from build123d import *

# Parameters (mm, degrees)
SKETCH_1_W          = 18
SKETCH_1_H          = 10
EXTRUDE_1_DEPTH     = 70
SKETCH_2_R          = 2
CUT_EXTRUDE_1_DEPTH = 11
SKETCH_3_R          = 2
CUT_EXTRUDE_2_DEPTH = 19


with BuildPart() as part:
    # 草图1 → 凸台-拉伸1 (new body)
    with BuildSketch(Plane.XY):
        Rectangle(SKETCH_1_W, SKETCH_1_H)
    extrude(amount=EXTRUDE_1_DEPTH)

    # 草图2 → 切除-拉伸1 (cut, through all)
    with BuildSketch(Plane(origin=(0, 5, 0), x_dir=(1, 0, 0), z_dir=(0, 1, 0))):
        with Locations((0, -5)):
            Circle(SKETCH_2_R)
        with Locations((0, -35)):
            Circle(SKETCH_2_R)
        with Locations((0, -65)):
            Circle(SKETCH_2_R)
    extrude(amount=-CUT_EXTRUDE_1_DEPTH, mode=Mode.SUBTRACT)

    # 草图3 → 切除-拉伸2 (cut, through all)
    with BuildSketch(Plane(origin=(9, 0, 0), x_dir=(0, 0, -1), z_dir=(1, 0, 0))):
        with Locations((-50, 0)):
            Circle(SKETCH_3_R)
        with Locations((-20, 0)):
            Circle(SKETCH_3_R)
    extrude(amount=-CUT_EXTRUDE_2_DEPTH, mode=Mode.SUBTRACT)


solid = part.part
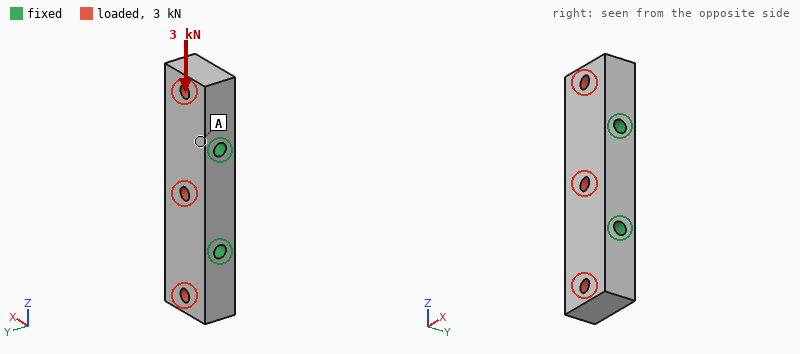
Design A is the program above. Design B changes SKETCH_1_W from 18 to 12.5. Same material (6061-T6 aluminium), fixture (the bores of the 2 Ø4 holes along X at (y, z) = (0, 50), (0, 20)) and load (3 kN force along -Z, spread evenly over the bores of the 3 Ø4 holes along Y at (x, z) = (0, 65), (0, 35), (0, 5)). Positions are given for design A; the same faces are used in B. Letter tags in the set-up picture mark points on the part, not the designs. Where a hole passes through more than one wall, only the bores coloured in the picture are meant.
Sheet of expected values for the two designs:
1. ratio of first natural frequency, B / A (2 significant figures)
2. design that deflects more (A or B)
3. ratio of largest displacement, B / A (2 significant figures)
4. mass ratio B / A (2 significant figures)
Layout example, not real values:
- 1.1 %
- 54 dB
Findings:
- 1.0
- B
- 1.2
- 0.68
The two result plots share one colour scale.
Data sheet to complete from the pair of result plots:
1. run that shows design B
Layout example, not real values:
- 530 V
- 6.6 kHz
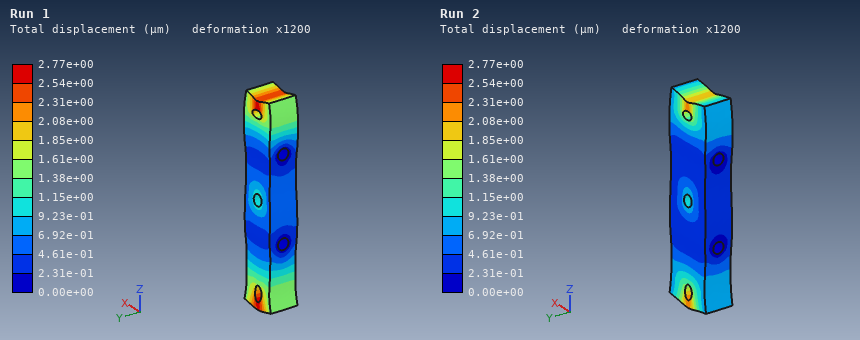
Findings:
- Run 1
